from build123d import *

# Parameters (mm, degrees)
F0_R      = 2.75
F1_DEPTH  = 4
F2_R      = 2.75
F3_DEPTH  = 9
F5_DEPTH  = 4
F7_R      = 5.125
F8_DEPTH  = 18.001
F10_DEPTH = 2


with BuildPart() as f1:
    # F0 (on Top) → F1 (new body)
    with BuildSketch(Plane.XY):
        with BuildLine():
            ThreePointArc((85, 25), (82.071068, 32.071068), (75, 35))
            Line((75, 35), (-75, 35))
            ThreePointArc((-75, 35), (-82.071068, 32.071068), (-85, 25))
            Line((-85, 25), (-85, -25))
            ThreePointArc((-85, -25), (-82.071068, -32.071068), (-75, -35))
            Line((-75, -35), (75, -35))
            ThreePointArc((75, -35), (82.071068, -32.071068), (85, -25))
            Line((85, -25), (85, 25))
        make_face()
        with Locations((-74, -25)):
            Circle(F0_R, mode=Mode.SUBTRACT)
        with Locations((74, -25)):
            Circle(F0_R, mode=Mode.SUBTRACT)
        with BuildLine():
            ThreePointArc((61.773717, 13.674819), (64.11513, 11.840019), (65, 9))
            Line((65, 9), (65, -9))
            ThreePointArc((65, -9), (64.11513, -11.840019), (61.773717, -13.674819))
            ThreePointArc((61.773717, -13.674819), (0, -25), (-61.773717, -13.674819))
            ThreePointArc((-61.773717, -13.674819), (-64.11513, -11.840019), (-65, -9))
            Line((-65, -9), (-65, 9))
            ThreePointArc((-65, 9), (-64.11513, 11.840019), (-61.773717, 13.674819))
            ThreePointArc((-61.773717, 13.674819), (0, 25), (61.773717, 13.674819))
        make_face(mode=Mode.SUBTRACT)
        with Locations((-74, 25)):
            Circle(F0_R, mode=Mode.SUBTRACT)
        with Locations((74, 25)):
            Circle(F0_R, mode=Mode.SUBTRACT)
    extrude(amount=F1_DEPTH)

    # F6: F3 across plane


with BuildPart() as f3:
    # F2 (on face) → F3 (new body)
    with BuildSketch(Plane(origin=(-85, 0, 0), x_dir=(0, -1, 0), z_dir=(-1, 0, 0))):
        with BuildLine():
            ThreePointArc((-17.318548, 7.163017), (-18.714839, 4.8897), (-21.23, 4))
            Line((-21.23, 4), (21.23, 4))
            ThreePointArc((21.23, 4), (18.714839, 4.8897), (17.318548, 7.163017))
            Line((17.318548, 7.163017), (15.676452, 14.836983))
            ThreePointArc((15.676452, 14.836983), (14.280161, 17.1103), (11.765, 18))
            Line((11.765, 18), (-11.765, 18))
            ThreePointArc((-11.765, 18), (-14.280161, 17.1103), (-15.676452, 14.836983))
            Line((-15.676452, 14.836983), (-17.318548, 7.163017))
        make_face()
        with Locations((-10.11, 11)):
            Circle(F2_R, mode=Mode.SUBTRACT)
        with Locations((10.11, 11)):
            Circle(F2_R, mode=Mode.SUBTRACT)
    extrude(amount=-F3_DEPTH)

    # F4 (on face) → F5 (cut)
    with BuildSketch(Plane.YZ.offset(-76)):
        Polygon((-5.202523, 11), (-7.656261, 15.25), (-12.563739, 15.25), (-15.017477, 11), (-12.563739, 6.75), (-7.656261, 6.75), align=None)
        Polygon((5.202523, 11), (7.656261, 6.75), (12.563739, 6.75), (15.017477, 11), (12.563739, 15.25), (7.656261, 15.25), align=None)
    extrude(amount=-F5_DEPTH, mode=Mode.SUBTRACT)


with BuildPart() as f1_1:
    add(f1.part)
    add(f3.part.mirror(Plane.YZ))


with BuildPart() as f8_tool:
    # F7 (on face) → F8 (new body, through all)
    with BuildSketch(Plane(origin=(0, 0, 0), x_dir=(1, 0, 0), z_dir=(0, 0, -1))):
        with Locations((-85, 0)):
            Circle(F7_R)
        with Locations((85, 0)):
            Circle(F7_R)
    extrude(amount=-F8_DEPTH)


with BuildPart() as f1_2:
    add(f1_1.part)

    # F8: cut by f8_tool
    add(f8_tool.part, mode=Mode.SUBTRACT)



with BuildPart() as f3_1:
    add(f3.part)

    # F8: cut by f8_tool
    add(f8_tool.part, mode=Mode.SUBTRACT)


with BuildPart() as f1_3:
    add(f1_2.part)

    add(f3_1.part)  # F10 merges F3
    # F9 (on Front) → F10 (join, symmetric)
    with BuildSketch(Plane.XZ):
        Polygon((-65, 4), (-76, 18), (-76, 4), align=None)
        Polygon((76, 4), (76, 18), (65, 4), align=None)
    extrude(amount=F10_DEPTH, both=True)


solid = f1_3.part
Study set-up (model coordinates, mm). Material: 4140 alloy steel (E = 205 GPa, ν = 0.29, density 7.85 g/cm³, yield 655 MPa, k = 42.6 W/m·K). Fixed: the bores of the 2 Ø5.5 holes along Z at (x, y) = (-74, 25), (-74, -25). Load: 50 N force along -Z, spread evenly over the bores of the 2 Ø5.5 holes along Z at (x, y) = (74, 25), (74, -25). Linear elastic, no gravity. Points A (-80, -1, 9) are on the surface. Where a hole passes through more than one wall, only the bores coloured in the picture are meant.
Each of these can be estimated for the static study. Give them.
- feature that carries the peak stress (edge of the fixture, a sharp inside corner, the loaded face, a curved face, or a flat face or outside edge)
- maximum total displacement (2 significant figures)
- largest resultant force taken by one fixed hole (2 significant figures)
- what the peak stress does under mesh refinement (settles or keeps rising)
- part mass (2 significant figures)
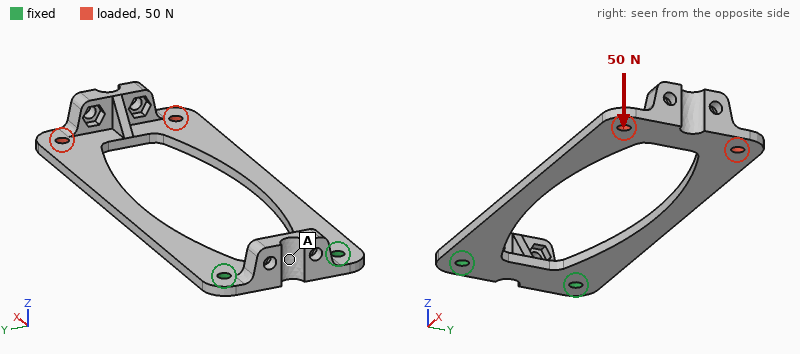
edge of the fixture
1.9 mm
36 N
keeps rising
240 g
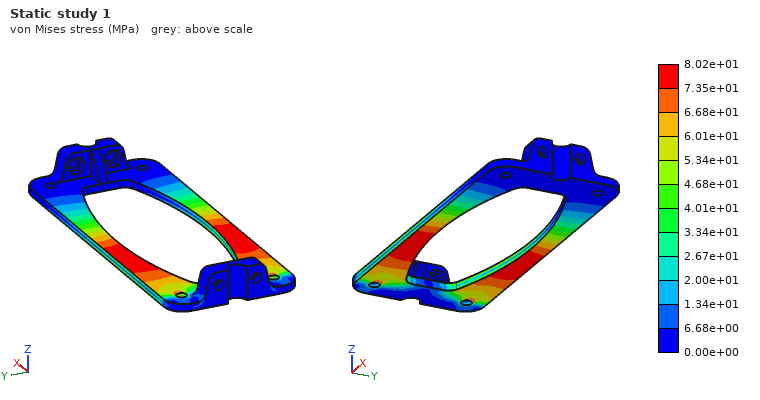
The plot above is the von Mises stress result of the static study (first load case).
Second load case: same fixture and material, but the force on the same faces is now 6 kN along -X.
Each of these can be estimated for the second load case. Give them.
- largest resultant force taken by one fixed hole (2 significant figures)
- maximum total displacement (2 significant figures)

3.0 kN
59 µm
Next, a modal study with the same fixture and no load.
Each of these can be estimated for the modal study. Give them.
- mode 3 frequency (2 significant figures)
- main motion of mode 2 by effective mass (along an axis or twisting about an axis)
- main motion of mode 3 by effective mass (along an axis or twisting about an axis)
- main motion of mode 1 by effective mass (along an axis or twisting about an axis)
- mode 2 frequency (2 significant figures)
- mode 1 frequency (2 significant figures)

700 Hz
twisting about X
along Y
along Z
410 Hz
91 Hz
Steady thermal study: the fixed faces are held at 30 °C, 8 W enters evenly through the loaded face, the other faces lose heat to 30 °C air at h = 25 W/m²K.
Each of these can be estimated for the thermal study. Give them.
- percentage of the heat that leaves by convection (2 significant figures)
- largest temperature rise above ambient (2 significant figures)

94 %
44 K
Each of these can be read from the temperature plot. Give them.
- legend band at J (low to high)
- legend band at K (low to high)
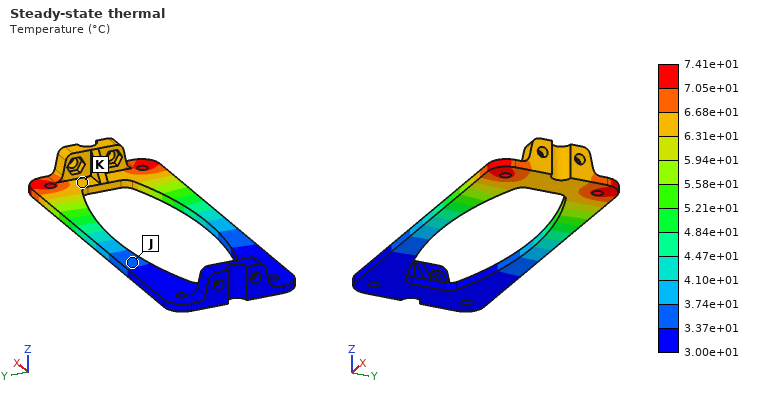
3.37e+01 to 3.74e+01 °C
6.31e+01 to 6.68e+01 °C
